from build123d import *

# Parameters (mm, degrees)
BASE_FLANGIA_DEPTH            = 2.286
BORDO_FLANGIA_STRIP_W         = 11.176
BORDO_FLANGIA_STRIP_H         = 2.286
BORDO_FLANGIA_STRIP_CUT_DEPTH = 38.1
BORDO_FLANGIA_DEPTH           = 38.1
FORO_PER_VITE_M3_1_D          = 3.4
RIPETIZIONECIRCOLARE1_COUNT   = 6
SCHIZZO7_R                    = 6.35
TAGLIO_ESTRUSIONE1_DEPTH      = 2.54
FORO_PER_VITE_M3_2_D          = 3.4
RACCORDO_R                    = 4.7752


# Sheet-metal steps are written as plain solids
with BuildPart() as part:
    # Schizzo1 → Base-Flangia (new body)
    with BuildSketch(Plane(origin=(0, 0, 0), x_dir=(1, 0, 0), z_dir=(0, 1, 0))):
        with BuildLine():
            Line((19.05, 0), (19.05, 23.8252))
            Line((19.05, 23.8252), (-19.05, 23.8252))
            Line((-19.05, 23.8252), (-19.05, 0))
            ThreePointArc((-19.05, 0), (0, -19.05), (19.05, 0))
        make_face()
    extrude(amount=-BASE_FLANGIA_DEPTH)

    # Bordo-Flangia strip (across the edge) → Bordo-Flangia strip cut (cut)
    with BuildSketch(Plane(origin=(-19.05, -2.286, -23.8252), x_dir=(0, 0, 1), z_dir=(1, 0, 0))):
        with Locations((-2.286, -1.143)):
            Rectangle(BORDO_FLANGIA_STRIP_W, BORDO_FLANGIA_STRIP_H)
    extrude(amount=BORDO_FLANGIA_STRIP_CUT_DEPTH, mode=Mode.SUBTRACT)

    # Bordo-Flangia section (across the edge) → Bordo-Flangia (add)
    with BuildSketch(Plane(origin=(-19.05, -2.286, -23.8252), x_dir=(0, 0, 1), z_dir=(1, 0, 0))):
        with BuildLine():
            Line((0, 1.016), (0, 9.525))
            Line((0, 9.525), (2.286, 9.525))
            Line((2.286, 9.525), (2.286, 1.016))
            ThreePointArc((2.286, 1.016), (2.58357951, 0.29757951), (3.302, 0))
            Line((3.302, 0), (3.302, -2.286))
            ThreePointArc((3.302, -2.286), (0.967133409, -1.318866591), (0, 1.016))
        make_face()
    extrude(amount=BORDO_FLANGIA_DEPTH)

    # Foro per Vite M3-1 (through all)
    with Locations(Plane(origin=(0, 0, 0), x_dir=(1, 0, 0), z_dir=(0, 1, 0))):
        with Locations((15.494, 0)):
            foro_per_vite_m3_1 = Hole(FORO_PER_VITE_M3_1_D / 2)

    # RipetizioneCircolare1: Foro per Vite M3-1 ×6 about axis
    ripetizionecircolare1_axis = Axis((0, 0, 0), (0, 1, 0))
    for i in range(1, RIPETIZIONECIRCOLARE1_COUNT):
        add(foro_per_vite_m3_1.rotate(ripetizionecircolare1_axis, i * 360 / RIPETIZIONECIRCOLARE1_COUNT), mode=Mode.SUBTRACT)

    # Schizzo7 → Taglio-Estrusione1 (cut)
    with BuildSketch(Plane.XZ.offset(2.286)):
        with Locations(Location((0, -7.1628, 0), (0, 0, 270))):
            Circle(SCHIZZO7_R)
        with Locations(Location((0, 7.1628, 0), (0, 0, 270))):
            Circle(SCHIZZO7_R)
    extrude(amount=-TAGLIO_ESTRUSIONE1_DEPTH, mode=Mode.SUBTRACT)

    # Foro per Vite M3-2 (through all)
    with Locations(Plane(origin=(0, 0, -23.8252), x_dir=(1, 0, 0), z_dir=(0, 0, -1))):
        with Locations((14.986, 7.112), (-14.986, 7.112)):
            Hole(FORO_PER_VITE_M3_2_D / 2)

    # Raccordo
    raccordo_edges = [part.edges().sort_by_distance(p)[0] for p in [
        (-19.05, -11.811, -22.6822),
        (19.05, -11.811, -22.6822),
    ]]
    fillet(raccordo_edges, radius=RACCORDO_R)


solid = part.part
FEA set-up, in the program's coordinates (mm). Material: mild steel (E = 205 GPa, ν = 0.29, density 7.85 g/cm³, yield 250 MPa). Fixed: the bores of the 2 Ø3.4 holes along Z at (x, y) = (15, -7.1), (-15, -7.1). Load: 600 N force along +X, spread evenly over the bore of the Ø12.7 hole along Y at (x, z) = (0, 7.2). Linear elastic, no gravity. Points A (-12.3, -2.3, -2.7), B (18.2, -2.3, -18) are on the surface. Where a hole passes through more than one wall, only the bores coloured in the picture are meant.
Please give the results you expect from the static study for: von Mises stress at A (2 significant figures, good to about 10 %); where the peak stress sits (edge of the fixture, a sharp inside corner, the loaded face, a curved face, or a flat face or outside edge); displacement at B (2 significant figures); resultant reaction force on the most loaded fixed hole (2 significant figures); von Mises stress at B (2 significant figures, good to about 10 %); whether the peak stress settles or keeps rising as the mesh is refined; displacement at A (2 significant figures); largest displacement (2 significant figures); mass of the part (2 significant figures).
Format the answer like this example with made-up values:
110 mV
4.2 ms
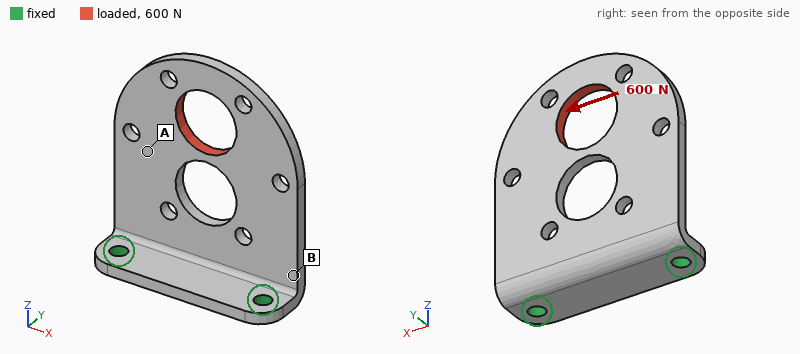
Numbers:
29 MPa
edge of the fixture
17 µm
670 N
84 MPa
keeps rising
30 µm
50 µm
26 g
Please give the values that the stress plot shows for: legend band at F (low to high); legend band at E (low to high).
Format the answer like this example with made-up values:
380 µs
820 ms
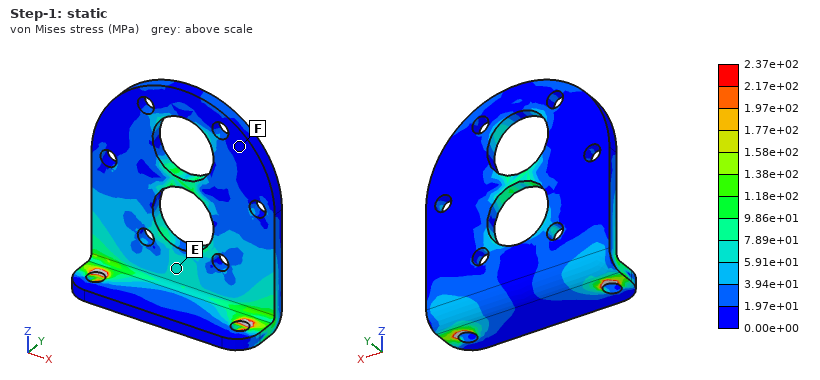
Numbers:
0.00e+00 to 1.97e+01 MPa
5.91e+01 to 7.89e+01 MPa
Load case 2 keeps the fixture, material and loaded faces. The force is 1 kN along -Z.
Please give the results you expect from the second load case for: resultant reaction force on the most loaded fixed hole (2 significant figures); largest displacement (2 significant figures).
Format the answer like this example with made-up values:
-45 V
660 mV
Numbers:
500 N
0.11 mm
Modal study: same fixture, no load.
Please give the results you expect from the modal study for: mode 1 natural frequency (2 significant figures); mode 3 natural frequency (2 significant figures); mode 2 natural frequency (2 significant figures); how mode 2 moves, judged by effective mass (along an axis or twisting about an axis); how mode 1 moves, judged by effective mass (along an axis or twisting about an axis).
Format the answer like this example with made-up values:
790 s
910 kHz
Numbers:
1100 Hz
5700 Hz
3000 Hz
twisting about Z
along Y
